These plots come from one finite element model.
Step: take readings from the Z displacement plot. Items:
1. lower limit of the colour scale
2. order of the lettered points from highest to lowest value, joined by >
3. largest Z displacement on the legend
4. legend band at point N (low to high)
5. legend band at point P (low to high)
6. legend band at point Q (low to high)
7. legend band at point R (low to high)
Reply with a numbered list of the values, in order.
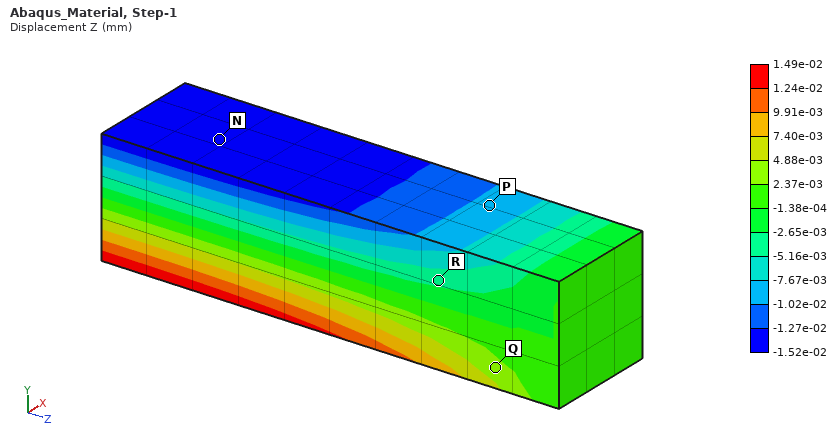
1. -1.52e-02 mm
2. Q > R > P > N
3. 1.49e-02 mm
4. -1.52e-02 to -1.27e-02 mm
5. -1.02e-02 to -7.67e-03 mm
6. 2.37e-03 to 4.88e-03 mm
7. -5.16e-03 to -2.65e-03 mm
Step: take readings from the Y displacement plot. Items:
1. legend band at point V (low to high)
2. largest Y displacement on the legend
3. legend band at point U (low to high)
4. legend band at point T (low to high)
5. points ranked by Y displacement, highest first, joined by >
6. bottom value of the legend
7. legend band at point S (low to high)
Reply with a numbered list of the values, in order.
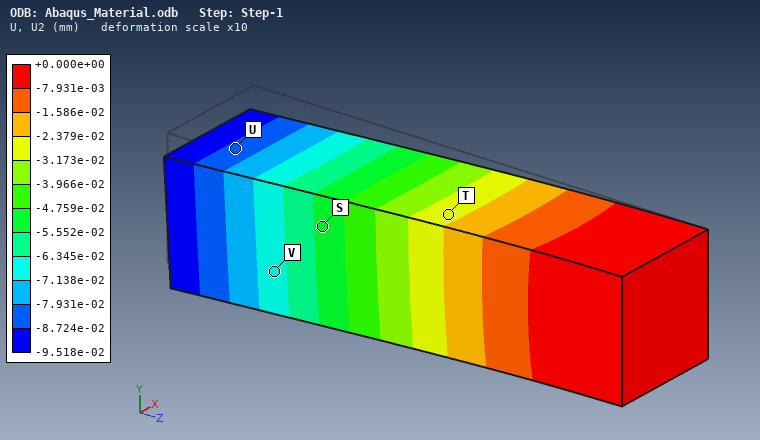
1. -7.138e-02 to -6.345e-02 mm
2. +0.000e+00 mm
3. -8.724e-02 to -7.931e-02 mm
4. -3.173e-02 to -2.379e-02 mm
5. T > S > V > U
6. -9.518e-02 mm
7. -5.552e-02 to -4.759e-02 mm
